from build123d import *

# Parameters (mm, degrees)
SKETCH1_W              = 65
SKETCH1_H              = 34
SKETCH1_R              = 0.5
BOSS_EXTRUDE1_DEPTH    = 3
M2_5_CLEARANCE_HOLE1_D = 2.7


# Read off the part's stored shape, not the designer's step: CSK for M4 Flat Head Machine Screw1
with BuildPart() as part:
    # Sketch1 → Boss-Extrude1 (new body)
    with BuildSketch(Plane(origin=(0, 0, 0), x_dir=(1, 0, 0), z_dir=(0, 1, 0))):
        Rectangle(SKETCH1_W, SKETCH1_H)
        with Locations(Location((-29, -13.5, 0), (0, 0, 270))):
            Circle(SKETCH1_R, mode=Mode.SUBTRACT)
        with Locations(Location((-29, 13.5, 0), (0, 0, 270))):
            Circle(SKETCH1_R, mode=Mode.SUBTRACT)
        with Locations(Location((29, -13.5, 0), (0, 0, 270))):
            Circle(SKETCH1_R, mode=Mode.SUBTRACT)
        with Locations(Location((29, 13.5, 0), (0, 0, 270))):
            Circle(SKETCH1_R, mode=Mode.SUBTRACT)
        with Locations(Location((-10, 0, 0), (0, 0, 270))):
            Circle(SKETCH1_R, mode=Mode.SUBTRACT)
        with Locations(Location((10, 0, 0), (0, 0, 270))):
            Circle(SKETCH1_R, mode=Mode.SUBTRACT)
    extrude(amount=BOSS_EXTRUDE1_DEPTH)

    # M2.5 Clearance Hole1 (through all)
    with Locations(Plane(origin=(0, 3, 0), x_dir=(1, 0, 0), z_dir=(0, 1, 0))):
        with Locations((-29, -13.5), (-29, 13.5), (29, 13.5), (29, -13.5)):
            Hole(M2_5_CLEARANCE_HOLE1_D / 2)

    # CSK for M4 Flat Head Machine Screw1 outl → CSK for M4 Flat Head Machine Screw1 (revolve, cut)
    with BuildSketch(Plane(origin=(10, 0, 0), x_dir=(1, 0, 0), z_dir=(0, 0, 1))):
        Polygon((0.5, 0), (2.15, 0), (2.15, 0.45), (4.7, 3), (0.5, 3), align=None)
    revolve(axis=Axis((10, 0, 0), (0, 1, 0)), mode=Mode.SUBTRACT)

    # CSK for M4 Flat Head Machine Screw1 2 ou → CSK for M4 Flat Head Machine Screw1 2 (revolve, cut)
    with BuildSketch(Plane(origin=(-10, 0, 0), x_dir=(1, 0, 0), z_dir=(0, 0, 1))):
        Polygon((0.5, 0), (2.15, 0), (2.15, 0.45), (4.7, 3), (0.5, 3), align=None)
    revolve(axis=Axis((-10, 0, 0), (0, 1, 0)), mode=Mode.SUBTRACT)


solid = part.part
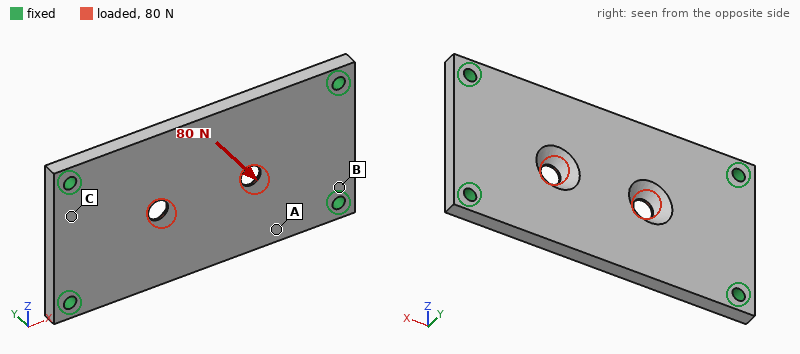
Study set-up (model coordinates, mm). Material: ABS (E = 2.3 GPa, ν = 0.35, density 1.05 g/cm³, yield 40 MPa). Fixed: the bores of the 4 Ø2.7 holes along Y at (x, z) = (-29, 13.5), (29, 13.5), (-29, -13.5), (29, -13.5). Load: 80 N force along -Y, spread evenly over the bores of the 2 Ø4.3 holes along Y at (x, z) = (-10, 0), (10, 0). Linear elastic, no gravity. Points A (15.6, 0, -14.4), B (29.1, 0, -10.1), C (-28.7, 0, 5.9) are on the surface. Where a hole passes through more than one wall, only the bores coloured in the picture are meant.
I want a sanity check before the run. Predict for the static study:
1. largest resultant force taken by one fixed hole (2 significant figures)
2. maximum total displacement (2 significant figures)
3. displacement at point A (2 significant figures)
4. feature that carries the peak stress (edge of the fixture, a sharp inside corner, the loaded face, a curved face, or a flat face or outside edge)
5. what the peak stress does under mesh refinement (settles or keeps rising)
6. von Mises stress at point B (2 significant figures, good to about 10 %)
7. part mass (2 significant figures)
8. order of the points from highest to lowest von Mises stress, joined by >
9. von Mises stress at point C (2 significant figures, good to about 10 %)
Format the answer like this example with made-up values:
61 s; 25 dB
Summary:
21 N; 0.48 mm; 0.21 mm; edge of the fixture; keeps rising; 7.6 MPa; 6.7 g; B > C > A; 4.3 MPa
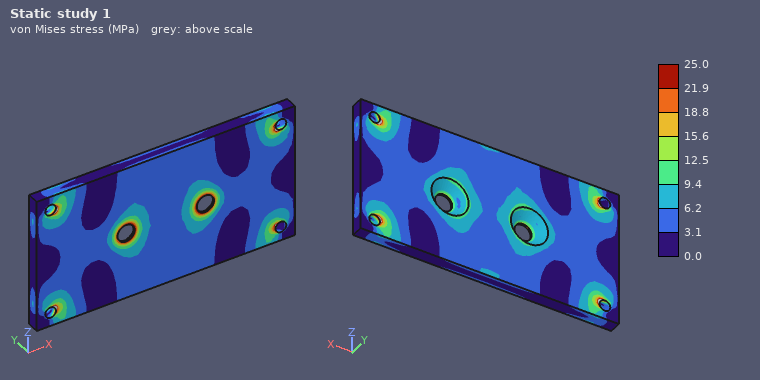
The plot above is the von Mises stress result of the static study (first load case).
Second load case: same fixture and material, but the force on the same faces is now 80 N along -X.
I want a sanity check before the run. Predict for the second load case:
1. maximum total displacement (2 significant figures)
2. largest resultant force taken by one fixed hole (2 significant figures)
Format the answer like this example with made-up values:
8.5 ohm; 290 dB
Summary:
16 µm; 21 N
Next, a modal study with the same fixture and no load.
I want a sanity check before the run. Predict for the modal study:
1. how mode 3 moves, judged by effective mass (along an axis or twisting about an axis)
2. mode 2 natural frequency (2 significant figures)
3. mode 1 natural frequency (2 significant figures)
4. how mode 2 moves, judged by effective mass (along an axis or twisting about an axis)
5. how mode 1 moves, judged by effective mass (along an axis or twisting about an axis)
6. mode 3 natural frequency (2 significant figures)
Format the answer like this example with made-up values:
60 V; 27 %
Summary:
twisting about Z; 2000 Hz; 1200 Hz; twisting about X; along Y; 3200 Hz
